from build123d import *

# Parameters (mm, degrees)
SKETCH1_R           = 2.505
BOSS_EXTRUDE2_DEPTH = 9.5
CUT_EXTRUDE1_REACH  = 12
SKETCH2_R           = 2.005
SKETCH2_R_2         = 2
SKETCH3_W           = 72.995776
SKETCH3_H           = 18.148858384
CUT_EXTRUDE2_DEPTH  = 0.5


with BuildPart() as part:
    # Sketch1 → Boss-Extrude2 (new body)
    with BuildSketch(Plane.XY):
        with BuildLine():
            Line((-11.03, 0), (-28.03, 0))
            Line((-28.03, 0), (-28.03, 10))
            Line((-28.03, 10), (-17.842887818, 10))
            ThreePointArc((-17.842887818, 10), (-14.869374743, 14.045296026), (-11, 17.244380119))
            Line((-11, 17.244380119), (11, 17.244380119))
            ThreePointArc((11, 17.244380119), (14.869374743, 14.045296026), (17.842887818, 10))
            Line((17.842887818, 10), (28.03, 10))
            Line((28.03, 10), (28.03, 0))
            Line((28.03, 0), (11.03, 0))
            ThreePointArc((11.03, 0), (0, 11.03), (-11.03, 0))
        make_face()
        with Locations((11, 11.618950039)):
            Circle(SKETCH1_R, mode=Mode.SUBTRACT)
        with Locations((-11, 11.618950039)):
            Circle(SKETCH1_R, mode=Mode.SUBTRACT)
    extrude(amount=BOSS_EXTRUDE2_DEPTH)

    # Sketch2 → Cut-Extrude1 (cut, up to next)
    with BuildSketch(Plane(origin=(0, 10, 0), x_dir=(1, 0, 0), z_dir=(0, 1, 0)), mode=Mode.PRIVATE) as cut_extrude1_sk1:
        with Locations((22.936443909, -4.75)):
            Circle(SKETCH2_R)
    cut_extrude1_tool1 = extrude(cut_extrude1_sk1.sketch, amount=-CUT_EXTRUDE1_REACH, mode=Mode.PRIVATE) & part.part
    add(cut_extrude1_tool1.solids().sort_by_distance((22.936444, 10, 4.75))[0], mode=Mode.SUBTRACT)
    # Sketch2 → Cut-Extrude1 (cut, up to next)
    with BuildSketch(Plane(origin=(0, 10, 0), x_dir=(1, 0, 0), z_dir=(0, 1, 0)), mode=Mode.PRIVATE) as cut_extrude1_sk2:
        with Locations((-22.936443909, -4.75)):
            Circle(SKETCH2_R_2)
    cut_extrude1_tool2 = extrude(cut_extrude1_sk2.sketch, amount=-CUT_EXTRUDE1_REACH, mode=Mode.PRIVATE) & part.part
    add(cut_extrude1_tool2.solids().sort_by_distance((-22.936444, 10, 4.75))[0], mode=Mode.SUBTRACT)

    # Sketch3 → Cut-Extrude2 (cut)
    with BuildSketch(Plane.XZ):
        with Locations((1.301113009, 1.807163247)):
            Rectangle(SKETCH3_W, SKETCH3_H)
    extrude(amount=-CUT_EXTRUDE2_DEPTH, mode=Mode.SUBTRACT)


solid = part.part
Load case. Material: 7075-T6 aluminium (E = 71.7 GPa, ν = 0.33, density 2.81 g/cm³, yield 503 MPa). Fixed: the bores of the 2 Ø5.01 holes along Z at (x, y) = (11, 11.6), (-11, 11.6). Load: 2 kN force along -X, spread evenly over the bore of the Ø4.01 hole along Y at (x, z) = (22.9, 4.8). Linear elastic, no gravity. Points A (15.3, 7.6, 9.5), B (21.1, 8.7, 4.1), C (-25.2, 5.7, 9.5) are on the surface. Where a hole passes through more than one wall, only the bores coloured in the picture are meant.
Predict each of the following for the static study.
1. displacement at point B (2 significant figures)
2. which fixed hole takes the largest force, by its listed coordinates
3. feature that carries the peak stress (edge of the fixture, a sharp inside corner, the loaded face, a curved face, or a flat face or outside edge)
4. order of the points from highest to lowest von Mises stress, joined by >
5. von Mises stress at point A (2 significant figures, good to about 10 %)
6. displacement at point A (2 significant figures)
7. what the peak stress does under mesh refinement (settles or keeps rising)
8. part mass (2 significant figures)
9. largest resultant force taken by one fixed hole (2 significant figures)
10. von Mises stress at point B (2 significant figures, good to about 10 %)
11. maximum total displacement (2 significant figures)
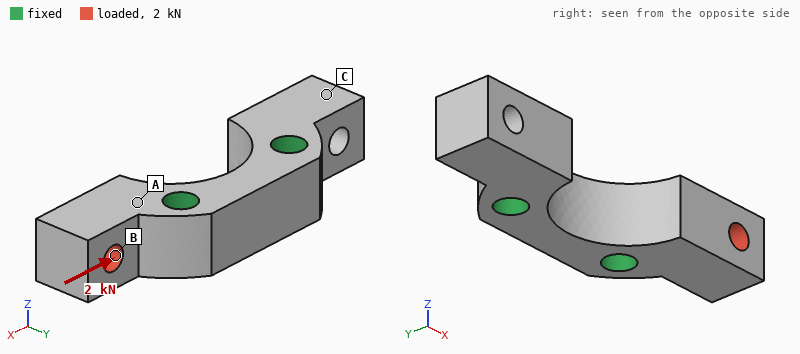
13 µm
(11, 11.6)
edge of the fixture
A > B > C
47 MPa
5.9 µm
keeps rising
13 g
2.0 kN
26 MPa
29 µm
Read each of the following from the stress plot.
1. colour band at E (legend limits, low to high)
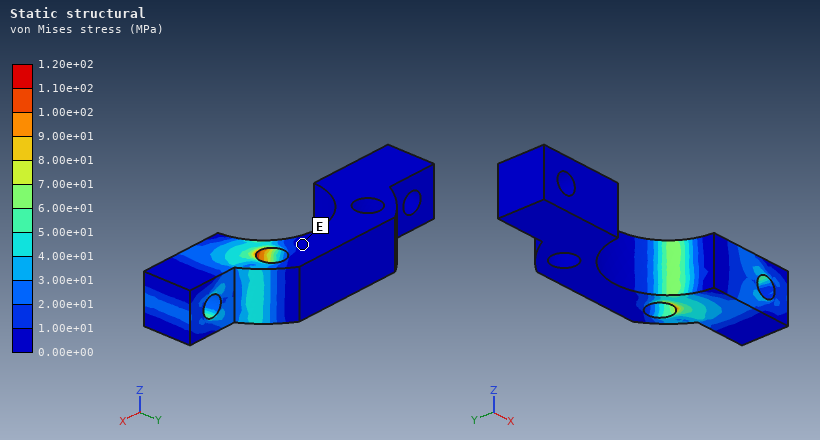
0.00e+00 to 1.00e+01 MPa
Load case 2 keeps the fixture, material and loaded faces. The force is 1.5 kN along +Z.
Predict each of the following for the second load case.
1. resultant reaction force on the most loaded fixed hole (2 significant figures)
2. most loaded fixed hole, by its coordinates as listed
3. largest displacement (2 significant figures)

1.5 kN
(11, 11.6)
52 µm
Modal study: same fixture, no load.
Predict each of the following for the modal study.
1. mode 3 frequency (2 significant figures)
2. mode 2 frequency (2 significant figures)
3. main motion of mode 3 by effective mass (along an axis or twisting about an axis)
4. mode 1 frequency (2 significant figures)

21 kHz
19 kHz
along Z
19 kHz
